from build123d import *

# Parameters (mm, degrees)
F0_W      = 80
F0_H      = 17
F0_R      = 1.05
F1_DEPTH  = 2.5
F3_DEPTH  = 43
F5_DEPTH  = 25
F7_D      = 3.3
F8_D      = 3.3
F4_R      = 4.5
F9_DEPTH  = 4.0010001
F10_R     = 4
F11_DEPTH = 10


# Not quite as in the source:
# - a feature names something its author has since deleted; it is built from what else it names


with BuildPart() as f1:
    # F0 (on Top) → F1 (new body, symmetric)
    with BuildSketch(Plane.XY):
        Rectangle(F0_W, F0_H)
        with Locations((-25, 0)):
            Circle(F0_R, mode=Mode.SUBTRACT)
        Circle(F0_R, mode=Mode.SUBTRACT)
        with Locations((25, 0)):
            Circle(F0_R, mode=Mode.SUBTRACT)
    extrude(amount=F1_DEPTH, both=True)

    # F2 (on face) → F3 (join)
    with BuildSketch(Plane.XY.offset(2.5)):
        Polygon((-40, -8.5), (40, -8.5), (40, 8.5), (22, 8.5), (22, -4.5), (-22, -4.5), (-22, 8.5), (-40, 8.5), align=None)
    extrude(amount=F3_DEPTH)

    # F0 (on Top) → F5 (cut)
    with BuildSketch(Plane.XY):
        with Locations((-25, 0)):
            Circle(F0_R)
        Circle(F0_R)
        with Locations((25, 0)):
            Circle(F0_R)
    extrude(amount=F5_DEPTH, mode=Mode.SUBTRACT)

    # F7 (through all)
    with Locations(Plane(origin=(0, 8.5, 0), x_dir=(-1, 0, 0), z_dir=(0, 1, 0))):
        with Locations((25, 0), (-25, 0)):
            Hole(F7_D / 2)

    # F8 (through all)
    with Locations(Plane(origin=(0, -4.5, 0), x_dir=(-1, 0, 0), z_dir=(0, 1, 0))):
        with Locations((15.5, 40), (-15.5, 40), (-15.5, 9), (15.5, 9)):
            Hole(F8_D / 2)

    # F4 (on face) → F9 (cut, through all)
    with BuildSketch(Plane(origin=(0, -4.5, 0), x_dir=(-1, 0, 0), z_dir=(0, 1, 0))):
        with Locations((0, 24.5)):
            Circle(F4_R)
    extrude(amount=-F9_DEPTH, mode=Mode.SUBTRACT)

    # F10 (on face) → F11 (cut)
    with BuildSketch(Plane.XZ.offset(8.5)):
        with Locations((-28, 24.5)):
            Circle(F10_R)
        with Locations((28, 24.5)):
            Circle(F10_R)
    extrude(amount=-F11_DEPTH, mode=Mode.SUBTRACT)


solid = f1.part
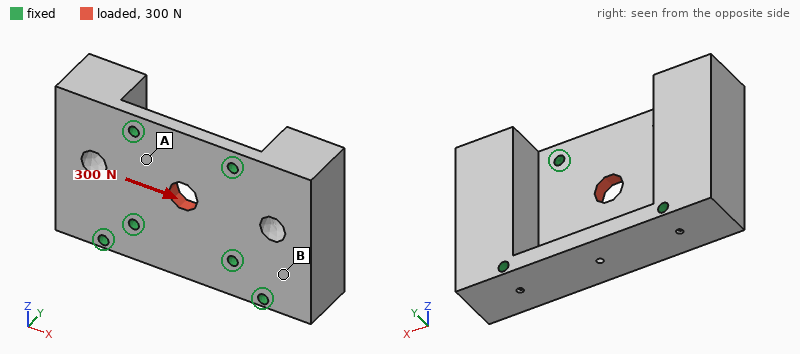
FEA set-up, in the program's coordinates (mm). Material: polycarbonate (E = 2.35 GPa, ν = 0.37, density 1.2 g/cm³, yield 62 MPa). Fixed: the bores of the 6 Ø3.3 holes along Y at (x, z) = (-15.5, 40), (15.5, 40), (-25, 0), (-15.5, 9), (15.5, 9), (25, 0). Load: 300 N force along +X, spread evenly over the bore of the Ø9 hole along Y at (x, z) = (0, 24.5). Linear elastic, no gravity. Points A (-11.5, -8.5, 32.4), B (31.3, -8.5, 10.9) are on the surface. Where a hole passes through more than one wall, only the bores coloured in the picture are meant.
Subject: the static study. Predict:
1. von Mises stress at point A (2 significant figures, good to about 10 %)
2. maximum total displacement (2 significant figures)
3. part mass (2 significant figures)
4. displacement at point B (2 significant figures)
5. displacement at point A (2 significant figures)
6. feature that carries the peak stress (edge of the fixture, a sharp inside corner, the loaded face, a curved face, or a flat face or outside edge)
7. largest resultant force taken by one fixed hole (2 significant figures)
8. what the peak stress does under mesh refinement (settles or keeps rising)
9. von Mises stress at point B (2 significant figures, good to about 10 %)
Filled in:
1.4 MPa
17 µm
47 g
2.9 µm
7.2 µm
edge of the fixture
78 N
keeps rising
0.29 MPa
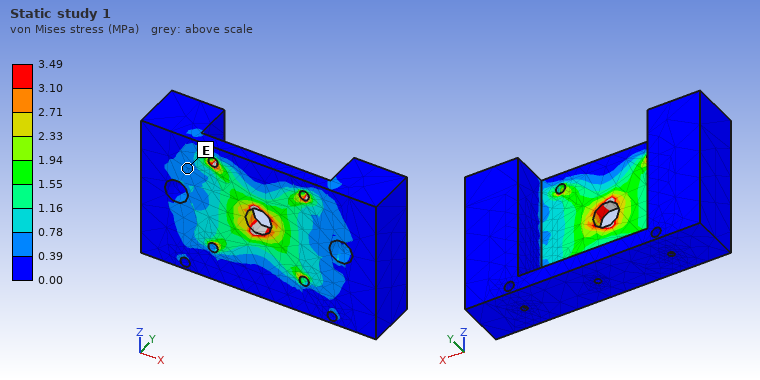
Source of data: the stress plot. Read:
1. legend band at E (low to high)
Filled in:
0.39 to 0.78 MPa
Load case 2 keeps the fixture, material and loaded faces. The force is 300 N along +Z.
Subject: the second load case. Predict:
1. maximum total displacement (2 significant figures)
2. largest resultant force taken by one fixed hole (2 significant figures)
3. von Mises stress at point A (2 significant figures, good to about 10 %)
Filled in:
21 µm
74 N
1.7 MPa
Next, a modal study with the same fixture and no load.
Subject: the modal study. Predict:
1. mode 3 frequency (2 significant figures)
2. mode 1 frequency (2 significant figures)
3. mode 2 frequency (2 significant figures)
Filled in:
4300 Hz
2100 Hz
2100 Hz
